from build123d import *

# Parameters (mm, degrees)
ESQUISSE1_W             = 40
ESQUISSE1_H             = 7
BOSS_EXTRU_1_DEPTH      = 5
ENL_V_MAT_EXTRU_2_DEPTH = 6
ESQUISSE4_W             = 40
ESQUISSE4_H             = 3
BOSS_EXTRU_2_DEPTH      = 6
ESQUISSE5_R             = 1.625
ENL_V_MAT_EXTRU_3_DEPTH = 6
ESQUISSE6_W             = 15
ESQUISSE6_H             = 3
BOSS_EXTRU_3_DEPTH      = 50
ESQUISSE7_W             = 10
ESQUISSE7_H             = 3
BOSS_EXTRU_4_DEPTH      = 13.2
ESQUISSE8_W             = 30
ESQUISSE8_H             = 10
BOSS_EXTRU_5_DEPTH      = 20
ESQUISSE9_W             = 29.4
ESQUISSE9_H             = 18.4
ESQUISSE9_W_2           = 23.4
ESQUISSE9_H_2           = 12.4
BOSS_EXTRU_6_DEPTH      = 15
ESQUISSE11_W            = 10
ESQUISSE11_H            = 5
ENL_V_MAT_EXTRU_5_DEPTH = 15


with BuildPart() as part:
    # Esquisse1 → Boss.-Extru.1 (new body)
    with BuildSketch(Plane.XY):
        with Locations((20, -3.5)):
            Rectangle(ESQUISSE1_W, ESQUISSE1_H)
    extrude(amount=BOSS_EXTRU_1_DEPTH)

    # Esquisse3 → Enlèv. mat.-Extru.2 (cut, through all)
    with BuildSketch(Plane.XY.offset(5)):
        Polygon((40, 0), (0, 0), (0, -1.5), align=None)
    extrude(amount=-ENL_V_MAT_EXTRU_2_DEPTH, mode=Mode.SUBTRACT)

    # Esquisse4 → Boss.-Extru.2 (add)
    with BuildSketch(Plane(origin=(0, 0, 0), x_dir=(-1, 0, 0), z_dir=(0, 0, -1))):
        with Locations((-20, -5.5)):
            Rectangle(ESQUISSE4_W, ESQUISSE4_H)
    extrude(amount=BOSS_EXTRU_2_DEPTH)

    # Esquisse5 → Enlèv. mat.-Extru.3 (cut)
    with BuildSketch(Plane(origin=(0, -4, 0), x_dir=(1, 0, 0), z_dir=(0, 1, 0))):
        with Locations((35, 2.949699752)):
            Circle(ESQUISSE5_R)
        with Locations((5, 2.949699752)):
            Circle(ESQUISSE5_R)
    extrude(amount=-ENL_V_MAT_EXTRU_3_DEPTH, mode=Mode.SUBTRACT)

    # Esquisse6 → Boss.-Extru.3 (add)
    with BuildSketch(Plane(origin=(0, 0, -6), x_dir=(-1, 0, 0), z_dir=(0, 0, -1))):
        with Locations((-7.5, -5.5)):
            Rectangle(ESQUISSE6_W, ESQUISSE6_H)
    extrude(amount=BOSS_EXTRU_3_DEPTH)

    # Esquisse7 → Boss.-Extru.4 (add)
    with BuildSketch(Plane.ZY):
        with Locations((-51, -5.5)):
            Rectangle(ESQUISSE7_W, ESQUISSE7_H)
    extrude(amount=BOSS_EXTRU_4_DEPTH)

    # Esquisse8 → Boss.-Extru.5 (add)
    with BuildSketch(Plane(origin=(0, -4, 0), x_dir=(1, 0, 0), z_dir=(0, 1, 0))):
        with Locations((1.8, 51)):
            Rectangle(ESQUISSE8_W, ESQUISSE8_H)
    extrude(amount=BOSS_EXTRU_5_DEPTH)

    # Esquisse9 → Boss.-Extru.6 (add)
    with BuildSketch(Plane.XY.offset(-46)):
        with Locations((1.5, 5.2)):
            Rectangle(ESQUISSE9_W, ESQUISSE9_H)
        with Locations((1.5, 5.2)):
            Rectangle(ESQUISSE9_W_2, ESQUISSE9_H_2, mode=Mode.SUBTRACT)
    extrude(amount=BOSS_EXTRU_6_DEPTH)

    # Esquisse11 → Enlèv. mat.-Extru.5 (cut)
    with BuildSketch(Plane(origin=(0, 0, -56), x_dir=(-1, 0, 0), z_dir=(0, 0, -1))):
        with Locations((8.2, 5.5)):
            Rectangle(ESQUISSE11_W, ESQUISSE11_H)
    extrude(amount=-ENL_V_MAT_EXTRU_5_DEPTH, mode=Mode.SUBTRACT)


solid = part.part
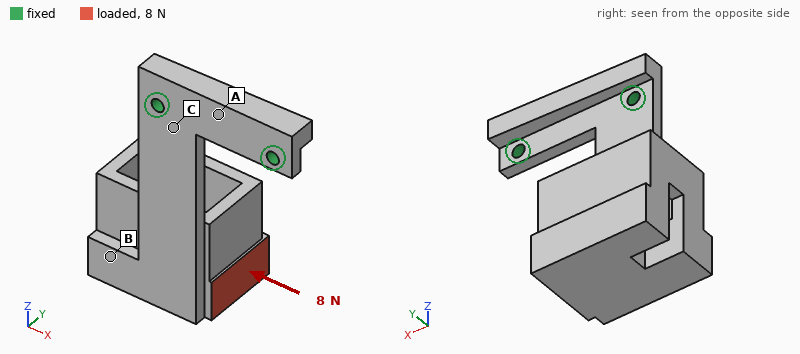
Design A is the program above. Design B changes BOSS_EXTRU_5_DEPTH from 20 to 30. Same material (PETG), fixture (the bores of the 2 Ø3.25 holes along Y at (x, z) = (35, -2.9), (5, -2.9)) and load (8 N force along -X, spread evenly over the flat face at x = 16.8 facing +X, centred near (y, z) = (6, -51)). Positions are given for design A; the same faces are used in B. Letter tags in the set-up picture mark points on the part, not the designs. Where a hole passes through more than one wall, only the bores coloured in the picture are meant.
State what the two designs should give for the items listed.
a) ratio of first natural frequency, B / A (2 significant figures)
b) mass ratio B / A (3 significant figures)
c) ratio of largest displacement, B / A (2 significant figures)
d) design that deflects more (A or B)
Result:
0.82
1.22
1.7
B
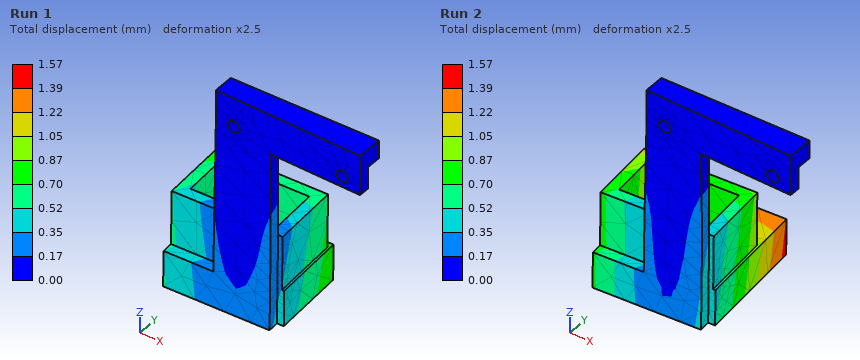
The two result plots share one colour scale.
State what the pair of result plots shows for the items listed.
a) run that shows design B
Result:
Run 2
